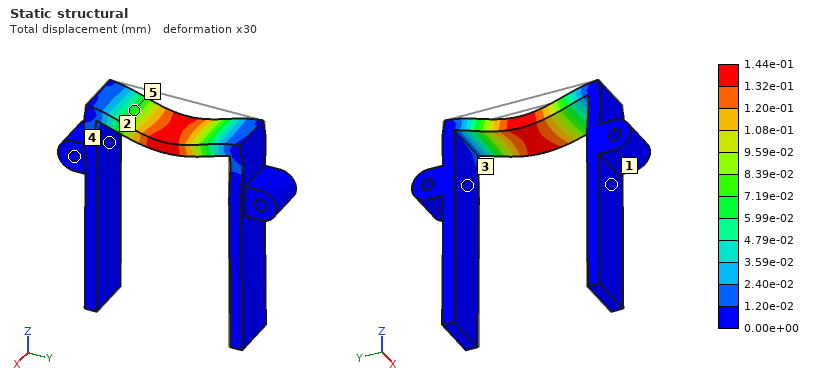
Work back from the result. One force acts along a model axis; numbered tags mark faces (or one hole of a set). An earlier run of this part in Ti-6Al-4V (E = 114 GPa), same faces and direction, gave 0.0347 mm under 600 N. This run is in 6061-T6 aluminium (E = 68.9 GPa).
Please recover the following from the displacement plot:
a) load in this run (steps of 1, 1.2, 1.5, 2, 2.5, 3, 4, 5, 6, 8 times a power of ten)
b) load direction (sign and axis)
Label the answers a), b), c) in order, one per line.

a) 1.5 kN
b) -Z
